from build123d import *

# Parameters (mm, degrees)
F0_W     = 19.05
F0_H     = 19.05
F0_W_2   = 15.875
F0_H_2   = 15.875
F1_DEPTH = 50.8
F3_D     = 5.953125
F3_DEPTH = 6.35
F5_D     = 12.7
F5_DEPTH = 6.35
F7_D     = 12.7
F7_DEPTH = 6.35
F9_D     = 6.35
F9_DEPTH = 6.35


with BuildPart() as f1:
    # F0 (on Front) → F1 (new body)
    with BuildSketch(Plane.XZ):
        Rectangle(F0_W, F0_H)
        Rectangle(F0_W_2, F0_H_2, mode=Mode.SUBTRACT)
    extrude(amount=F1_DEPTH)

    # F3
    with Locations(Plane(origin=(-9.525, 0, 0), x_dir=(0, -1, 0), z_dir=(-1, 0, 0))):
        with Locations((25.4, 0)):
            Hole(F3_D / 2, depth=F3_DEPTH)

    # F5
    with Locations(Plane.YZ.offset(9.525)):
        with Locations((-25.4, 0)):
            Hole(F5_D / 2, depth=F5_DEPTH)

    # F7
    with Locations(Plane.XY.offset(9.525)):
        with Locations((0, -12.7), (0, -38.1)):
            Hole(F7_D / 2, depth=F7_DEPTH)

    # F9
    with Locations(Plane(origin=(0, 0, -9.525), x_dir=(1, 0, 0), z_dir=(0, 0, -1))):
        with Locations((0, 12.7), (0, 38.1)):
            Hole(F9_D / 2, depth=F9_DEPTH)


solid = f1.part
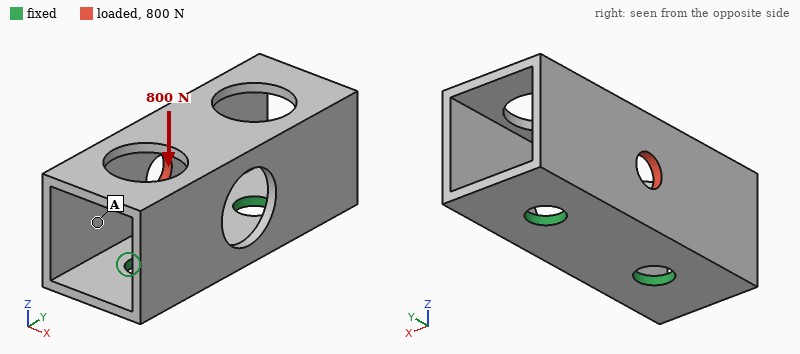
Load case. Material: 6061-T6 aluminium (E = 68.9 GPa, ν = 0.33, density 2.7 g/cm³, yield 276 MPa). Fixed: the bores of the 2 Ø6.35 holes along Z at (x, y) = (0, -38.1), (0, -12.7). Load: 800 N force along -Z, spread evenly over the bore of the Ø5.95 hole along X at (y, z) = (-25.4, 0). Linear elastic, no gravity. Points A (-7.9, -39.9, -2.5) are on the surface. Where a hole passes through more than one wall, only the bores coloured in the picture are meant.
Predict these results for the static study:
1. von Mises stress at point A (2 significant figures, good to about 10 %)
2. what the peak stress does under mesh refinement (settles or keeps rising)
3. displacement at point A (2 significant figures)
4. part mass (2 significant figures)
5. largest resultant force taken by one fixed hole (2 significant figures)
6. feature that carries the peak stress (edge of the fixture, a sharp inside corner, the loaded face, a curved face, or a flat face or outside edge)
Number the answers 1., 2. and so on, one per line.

1. 45 MPa
2. keeps rising
3. 0.090 mm
4. 13 g
5. 410 N
6. edge of the fixture
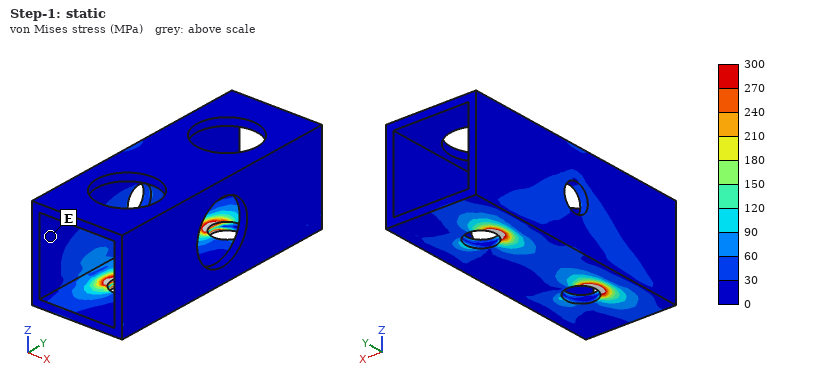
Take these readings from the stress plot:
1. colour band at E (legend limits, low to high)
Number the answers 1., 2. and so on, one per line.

1. 0 to 30 MPa
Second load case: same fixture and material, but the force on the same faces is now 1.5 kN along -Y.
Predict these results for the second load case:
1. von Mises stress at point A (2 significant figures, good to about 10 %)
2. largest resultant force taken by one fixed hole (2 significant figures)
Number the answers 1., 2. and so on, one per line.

1. 44 MPa
2. 950 N
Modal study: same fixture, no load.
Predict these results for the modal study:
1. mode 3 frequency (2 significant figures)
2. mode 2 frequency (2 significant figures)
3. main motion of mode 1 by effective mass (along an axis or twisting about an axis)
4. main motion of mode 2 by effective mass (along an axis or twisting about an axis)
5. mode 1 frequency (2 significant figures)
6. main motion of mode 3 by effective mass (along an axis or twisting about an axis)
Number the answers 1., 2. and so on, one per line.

1. 6700 Hz
2. 5700 Hz
3. along X
4. along Y
5. 2400 Hz
6. twisting about Z
